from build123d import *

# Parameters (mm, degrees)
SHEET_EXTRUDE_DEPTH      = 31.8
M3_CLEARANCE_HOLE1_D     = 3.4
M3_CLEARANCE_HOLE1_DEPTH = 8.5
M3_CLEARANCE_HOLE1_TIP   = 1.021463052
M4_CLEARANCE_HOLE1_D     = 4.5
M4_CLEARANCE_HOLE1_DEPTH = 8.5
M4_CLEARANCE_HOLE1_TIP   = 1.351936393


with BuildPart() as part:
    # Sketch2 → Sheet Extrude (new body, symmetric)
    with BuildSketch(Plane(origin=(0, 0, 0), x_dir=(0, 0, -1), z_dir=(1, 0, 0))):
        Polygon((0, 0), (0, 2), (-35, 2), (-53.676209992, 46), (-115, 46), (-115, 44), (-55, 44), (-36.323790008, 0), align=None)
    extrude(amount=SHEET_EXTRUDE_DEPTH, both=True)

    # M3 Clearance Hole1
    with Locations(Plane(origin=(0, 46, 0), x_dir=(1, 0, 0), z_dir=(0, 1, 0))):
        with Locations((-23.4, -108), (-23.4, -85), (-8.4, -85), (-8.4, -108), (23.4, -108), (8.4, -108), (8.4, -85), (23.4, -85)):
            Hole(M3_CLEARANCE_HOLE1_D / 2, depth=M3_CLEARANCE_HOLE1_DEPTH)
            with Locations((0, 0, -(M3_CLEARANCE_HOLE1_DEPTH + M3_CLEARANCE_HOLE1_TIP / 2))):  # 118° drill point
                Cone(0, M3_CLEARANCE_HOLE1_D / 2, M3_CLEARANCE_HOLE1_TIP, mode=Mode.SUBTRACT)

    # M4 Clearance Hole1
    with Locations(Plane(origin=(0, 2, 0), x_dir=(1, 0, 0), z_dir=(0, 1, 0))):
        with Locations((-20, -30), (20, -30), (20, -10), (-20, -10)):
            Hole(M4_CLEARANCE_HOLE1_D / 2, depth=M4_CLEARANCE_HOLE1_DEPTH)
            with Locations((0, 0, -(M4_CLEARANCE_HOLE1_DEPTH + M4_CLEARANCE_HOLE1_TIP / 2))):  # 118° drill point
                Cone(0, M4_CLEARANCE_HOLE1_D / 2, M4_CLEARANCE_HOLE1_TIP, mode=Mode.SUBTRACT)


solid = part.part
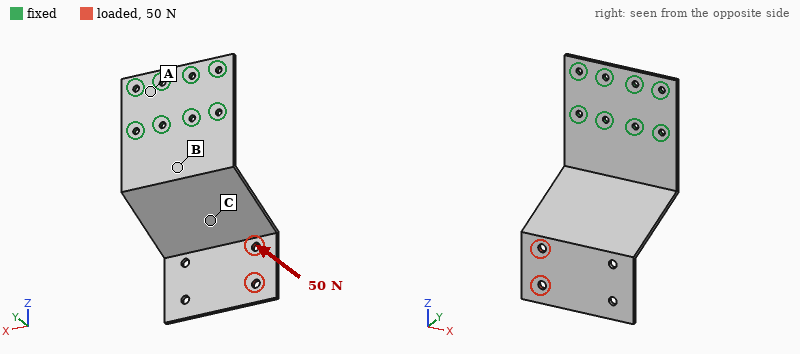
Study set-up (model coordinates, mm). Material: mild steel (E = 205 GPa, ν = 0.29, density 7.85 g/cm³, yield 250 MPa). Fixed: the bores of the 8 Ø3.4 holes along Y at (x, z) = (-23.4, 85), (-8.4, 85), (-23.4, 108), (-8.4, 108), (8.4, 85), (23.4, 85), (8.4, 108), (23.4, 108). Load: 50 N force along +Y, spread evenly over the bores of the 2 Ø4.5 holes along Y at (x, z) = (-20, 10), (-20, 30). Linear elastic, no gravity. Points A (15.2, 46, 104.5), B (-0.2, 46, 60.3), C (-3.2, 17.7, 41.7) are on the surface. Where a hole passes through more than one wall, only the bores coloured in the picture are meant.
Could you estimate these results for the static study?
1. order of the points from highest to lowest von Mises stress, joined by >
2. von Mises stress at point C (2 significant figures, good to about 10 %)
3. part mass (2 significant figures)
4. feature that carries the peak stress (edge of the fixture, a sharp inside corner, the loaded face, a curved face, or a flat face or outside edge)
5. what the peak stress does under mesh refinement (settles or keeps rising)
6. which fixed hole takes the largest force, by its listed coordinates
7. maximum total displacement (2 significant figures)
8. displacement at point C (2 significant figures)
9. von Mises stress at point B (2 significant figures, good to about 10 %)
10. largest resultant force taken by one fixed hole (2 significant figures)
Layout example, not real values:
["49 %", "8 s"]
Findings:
["B > C > A", "26 MPa", "140 g", "edge of the fixture", "keeps rising", "(-23.4, 85)", "1.1 mm", "0.40 mm", "45 MPa", "33 N"]
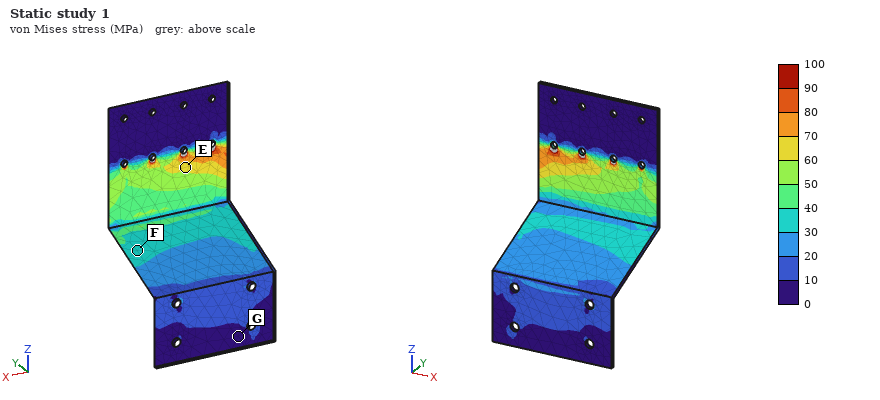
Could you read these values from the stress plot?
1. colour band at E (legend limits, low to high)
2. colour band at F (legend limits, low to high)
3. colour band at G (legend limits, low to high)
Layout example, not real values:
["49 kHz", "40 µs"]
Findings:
["60 to 70 MPa", "30 to 40 MPa", "0 to 10 MPa"]
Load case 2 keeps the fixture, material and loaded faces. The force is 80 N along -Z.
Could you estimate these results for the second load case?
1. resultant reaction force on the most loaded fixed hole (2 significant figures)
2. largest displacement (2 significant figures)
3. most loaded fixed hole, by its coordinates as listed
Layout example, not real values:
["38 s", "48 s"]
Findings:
["39 N", "1.6 mm", "(-23.4, 85)"]
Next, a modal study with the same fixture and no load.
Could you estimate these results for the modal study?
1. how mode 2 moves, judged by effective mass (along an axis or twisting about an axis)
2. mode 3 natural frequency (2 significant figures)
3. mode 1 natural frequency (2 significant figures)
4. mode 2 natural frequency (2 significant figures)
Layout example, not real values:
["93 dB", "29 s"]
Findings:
["along X", "590 Hz", "160 Hz", "490 Hz"]
